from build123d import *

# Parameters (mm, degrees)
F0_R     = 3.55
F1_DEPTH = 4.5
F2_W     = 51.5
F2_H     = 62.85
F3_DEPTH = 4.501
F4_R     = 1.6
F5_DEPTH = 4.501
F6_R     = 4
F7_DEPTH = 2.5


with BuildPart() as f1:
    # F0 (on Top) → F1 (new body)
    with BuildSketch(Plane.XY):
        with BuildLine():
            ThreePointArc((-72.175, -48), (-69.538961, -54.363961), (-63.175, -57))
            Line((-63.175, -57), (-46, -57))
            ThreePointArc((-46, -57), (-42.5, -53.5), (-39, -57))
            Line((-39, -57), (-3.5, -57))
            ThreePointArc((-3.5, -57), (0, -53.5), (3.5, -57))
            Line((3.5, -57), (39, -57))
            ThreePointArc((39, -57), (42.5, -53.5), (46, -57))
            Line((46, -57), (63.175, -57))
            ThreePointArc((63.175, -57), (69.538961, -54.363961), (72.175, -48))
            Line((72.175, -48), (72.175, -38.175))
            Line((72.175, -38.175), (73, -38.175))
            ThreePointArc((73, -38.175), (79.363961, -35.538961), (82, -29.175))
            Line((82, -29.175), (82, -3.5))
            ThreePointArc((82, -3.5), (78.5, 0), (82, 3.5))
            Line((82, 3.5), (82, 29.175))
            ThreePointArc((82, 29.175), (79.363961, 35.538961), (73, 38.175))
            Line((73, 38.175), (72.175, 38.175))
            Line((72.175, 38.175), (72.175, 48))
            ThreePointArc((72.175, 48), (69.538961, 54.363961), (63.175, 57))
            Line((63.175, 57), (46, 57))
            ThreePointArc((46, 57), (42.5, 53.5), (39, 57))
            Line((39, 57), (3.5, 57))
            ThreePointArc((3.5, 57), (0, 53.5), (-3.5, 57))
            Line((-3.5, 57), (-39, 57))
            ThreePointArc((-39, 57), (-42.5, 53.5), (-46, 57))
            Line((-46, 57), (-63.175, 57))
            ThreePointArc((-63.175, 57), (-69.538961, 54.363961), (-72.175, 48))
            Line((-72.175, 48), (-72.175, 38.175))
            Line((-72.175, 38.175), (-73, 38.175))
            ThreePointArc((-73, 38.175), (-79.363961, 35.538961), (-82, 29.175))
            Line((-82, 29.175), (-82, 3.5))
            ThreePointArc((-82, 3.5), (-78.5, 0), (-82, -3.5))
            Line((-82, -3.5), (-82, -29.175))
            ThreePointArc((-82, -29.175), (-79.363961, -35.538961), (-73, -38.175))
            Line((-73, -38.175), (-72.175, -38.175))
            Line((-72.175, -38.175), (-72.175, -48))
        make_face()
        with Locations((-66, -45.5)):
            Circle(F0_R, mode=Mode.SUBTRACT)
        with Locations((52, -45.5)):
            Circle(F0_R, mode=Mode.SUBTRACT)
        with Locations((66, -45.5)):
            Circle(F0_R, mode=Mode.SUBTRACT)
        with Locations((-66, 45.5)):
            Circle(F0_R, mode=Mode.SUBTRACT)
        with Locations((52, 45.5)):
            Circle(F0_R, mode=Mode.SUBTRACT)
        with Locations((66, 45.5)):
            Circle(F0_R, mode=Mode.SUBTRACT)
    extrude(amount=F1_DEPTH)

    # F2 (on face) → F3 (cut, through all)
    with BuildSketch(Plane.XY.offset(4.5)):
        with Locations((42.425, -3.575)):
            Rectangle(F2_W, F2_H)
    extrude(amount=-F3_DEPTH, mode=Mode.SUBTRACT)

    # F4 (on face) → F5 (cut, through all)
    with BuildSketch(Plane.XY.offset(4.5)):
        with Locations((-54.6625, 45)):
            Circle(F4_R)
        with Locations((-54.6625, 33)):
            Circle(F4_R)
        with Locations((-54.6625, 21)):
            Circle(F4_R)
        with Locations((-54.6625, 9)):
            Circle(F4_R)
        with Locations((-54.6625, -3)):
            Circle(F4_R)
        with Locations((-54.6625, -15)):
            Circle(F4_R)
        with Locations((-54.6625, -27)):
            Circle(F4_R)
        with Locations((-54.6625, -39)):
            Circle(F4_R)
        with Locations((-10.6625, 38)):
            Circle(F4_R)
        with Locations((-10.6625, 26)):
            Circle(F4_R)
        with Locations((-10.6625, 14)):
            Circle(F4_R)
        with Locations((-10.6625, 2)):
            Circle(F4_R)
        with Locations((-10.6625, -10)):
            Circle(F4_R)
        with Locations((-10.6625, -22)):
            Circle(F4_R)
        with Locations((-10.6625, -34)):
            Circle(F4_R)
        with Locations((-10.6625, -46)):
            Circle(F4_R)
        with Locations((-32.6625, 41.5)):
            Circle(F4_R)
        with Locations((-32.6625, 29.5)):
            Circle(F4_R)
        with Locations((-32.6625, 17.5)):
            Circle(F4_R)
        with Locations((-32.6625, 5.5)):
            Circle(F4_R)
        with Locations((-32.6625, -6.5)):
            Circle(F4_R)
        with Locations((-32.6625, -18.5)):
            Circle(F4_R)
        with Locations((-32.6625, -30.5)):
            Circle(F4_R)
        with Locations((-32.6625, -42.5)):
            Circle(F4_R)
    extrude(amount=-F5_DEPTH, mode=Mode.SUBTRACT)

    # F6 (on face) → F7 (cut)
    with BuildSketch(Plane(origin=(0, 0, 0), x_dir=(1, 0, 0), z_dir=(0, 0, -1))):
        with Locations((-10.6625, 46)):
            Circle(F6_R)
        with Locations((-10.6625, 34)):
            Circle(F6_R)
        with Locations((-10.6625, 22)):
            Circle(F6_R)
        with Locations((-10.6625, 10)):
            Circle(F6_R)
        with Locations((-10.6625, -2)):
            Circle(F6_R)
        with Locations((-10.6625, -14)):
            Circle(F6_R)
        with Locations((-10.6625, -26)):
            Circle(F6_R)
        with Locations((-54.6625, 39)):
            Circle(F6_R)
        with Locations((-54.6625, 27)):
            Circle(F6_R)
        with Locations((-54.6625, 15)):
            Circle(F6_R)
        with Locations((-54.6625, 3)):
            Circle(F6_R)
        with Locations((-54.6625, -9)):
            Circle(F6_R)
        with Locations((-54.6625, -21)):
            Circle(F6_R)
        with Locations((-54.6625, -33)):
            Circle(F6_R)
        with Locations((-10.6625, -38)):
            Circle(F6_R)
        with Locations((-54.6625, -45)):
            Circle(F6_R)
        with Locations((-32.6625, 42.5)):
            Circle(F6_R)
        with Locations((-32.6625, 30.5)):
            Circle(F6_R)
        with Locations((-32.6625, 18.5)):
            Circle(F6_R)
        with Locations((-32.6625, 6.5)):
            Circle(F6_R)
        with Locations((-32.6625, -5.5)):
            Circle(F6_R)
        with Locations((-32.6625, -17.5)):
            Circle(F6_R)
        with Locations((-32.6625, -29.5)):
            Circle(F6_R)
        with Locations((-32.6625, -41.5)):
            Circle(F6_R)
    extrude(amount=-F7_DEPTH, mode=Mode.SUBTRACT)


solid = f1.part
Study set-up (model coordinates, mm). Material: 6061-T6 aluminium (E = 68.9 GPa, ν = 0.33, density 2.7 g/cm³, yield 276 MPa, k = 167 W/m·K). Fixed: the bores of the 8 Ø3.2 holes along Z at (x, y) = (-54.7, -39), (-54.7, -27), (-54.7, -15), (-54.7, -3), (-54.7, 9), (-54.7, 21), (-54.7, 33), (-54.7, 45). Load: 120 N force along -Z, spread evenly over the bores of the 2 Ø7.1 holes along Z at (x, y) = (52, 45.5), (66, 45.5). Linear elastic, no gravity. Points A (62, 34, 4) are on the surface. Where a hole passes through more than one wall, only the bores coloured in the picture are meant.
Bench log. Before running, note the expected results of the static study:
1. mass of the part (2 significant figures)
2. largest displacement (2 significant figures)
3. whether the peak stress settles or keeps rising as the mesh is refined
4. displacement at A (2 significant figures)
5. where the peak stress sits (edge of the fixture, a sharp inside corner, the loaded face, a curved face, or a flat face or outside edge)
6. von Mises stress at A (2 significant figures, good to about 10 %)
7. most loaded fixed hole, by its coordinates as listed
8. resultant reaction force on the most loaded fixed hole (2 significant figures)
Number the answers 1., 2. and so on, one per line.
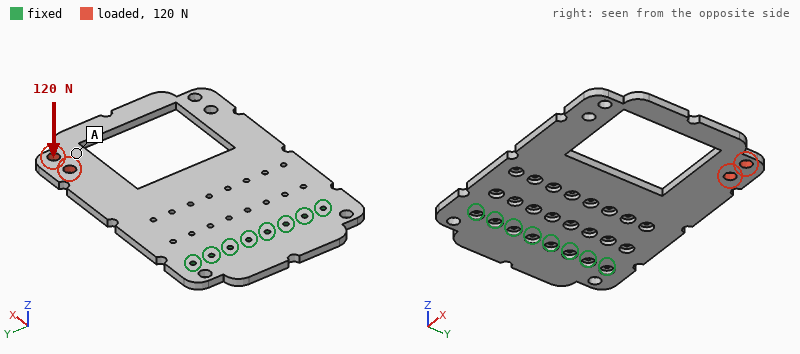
1. 160 g
2. 2.4 mm
3. keeps rising
4. 1.9 mm
5. edge of the fixture
6. 17 MPa
7. (-54.7, -39)
8. 130 N
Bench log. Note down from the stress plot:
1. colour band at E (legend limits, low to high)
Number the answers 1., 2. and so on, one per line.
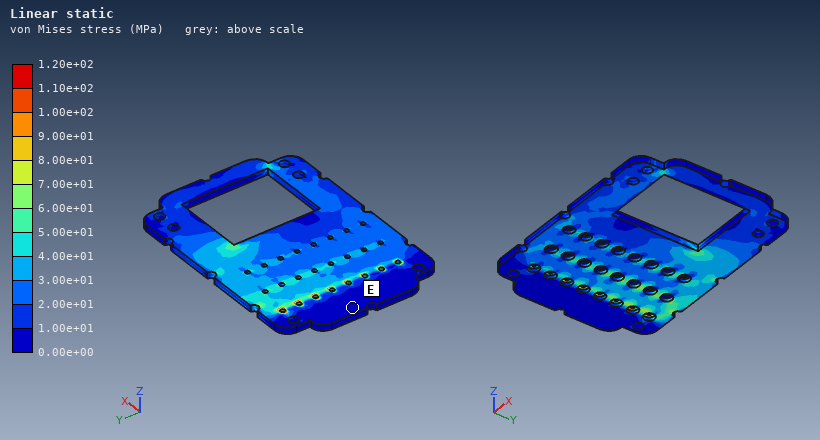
1. 0.00e+00 to 1.00e+01 MPa
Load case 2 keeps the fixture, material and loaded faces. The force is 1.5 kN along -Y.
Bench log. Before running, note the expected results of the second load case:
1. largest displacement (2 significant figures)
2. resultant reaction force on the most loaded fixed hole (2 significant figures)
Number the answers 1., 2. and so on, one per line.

1. 0.20 mm
2. 1.5 kN
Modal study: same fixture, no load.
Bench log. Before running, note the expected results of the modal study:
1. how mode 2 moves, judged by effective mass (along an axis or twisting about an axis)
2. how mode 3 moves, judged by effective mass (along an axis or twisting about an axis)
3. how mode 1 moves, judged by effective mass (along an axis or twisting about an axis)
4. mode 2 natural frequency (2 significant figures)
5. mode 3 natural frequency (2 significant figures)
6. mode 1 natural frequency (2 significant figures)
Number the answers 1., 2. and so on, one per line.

1. twisting about X
2. along Z
3. along Z
4. 510 Hz
5. 950 Hz
6. 210 Hz
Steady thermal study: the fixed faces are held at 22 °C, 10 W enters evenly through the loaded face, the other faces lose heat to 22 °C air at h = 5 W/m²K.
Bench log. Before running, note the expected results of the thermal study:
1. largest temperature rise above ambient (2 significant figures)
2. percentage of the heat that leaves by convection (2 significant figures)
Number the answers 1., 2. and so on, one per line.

1. 33 K
2. 13 %
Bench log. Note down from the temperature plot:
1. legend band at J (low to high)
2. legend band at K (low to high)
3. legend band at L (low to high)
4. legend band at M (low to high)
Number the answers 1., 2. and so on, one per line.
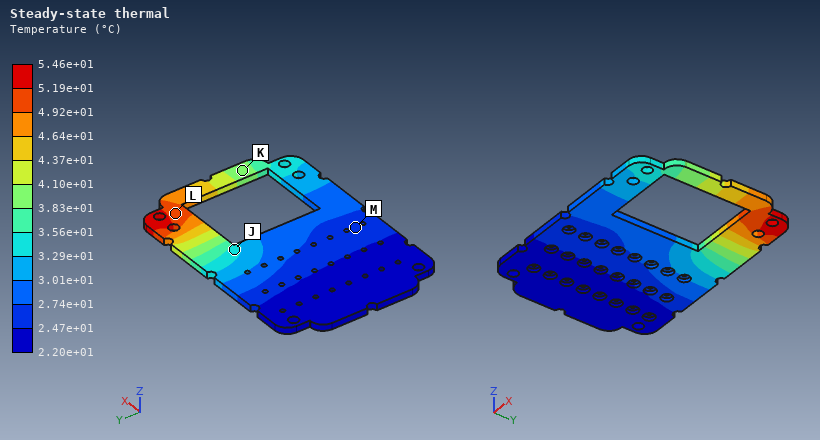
1. 3.29e+01 to 3.56e+01 °C
2. 3.83e+01 to 4.10e+01 °C
3. 4.92e+01 to 5.19e+01 °C
4. 2.47e+01 to 2.74e+01 °C
